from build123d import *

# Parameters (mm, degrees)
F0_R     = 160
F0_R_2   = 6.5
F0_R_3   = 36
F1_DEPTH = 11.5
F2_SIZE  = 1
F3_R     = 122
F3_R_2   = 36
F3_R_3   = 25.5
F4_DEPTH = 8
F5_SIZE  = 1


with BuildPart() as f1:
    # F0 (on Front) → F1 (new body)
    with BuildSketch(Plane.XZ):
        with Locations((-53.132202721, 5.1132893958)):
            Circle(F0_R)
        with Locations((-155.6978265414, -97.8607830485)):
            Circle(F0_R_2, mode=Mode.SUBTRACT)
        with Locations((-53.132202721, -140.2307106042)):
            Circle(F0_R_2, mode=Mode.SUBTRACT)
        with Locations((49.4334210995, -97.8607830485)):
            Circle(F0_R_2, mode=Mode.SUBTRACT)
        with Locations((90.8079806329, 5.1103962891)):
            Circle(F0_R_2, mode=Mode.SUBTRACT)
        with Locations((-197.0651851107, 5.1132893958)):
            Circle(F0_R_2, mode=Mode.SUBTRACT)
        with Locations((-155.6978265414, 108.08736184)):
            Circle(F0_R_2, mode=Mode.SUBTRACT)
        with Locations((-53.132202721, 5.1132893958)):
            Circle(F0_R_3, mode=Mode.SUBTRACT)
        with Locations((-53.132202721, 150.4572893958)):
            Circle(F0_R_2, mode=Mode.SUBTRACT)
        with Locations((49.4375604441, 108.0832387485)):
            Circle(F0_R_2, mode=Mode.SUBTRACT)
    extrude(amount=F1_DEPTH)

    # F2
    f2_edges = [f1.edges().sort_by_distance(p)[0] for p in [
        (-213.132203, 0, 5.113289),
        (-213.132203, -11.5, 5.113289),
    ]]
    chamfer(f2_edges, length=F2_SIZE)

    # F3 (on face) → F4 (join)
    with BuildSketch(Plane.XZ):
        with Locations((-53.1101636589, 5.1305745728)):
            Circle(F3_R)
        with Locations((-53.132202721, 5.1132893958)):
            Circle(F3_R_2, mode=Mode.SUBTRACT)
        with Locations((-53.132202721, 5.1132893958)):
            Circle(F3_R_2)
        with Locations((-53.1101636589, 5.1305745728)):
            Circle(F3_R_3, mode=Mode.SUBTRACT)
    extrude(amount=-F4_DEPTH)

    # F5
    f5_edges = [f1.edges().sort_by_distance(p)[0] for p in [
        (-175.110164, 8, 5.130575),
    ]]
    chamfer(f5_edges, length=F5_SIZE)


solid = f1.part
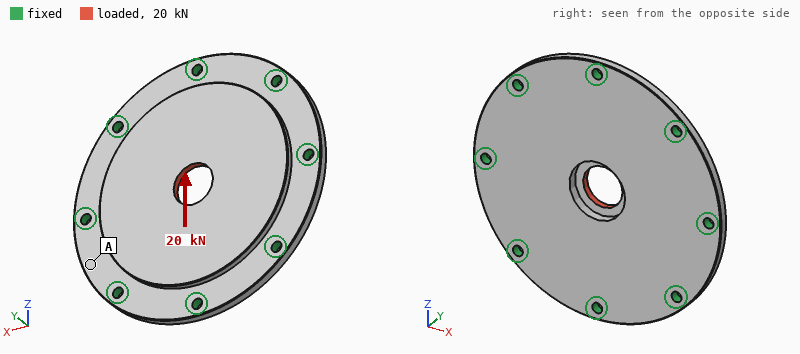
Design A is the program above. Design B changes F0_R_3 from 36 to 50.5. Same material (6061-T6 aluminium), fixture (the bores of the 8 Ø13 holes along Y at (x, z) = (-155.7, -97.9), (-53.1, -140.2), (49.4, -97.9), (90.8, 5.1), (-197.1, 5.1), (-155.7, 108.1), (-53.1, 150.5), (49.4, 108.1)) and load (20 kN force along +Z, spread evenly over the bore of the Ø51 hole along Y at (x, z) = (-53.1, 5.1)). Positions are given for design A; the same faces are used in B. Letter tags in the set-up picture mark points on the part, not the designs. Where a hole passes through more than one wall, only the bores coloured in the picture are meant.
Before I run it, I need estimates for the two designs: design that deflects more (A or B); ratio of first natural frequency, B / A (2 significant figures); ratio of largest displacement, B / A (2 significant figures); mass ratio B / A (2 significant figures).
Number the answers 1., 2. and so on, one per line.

1. B
2. 1.0
3. 1.2
4. 0.96
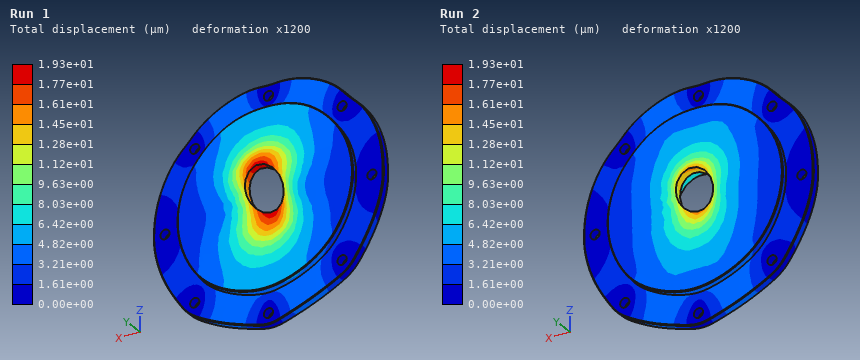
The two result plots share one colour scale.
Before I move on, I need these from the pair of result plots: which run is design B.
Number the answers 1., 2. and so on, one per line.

1. Run 1
